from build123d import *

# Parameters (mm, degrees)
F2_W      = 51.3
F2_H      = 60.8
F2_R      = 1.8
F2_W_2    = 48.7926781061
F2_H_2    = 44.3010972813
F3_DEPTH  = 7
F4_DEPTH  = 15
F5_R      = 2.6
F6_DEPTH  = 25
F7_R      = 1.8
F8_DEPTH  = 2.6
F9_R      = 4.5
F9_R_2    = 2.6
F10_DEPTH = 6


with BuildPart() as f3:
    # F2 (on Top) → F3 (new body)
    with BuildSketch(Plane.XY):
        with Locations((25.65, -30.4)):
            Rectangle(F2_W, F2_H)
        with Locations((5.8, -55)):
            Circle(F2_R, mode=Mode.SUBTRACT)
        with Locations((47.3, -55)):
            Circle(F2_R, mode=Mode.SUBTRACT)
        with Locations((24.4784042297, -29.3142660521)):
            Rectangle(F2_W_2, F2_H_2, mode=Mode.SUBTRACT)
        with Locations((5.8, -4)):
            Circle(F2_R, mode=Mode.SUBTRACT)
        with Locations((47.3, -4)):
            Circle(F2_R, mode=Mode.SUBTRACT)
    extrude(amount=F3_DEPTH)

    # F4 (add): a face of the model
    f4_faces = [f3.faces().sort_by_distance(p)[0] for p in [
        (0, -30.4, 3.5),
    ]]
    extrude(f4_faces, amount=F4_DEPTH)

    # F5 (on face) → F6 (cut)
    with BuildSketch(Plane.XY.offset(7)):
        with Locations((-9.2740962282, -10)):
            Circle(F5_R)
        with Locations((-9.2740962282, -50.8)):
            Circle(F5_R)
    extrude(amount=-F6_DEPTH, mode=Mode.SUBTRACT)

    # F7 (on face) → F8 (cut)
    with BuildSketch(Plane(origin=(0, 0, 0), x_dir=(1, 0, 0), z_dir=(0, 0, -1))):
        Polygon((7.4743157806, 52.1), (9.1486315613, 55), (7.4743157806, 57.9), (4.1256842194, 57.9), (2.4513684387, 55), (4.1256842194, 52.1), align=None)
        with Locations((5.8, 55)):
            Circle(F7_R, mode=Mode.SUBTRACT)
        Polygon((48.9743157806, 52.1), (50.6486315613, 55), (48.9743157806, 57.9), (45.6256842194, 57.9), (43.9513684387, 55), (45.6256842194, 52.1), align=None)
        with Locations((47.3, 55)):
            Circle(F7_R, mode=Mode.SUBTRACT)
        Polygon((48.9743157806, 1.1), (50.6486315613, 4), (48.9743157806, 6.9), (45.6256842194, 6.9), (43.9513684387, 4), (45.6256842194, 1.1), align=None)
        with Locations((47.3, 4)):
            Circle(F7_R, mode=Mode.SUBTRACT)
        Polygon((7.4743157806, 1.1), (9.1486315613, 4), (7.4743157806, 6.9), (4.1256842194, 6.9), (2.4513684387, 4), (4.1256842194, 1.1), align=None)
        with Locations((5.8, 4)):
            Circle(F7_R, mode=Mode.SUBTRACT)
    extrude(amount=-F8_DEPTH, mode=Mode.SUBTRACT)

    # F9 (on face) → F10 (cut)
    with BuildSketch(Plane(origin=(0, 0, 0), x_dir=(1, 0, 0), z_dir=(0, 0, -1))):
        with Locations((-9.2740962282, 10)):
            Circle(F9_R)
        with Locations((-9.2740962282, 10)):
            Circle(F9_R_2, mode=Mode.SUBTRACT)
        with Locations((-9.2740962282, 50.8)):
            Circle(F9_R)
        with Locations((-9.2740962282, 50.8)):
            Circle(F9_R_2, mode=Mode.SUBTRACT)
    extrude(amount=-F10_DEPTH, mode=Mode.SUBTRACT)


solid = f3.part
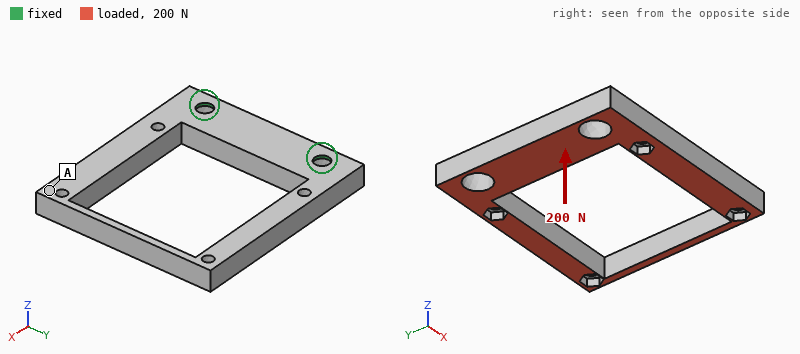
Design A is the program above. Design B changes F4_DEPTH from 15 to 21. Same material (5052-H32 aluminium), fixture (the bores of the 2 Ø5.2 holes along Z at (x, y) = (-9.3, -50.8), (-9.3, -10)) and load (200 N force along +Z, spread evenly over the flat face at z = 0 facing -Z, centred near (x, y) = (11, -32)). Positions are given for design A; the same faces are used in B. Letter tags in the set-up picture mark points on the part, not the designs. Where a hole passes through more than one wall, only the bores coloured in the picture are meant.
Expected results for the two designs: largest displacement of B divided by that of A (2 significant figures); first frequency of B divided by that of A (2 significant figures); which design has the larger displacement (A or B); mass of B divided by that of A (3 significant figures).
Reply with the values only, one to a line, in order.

0.74
1.0
A
1.22
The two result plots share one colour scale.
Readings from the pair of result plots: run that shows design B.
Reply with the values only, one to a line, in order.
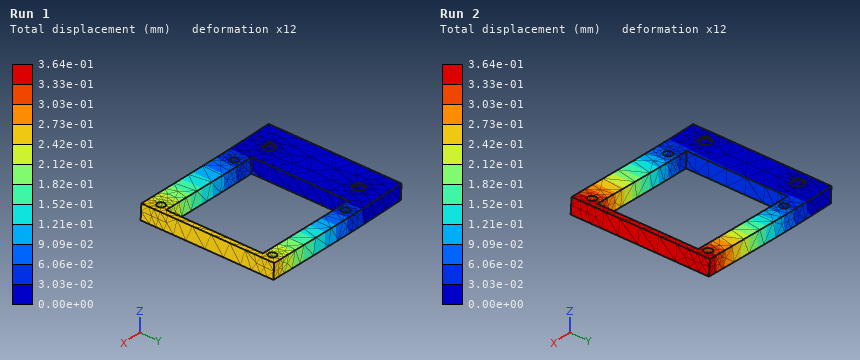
Run 1
